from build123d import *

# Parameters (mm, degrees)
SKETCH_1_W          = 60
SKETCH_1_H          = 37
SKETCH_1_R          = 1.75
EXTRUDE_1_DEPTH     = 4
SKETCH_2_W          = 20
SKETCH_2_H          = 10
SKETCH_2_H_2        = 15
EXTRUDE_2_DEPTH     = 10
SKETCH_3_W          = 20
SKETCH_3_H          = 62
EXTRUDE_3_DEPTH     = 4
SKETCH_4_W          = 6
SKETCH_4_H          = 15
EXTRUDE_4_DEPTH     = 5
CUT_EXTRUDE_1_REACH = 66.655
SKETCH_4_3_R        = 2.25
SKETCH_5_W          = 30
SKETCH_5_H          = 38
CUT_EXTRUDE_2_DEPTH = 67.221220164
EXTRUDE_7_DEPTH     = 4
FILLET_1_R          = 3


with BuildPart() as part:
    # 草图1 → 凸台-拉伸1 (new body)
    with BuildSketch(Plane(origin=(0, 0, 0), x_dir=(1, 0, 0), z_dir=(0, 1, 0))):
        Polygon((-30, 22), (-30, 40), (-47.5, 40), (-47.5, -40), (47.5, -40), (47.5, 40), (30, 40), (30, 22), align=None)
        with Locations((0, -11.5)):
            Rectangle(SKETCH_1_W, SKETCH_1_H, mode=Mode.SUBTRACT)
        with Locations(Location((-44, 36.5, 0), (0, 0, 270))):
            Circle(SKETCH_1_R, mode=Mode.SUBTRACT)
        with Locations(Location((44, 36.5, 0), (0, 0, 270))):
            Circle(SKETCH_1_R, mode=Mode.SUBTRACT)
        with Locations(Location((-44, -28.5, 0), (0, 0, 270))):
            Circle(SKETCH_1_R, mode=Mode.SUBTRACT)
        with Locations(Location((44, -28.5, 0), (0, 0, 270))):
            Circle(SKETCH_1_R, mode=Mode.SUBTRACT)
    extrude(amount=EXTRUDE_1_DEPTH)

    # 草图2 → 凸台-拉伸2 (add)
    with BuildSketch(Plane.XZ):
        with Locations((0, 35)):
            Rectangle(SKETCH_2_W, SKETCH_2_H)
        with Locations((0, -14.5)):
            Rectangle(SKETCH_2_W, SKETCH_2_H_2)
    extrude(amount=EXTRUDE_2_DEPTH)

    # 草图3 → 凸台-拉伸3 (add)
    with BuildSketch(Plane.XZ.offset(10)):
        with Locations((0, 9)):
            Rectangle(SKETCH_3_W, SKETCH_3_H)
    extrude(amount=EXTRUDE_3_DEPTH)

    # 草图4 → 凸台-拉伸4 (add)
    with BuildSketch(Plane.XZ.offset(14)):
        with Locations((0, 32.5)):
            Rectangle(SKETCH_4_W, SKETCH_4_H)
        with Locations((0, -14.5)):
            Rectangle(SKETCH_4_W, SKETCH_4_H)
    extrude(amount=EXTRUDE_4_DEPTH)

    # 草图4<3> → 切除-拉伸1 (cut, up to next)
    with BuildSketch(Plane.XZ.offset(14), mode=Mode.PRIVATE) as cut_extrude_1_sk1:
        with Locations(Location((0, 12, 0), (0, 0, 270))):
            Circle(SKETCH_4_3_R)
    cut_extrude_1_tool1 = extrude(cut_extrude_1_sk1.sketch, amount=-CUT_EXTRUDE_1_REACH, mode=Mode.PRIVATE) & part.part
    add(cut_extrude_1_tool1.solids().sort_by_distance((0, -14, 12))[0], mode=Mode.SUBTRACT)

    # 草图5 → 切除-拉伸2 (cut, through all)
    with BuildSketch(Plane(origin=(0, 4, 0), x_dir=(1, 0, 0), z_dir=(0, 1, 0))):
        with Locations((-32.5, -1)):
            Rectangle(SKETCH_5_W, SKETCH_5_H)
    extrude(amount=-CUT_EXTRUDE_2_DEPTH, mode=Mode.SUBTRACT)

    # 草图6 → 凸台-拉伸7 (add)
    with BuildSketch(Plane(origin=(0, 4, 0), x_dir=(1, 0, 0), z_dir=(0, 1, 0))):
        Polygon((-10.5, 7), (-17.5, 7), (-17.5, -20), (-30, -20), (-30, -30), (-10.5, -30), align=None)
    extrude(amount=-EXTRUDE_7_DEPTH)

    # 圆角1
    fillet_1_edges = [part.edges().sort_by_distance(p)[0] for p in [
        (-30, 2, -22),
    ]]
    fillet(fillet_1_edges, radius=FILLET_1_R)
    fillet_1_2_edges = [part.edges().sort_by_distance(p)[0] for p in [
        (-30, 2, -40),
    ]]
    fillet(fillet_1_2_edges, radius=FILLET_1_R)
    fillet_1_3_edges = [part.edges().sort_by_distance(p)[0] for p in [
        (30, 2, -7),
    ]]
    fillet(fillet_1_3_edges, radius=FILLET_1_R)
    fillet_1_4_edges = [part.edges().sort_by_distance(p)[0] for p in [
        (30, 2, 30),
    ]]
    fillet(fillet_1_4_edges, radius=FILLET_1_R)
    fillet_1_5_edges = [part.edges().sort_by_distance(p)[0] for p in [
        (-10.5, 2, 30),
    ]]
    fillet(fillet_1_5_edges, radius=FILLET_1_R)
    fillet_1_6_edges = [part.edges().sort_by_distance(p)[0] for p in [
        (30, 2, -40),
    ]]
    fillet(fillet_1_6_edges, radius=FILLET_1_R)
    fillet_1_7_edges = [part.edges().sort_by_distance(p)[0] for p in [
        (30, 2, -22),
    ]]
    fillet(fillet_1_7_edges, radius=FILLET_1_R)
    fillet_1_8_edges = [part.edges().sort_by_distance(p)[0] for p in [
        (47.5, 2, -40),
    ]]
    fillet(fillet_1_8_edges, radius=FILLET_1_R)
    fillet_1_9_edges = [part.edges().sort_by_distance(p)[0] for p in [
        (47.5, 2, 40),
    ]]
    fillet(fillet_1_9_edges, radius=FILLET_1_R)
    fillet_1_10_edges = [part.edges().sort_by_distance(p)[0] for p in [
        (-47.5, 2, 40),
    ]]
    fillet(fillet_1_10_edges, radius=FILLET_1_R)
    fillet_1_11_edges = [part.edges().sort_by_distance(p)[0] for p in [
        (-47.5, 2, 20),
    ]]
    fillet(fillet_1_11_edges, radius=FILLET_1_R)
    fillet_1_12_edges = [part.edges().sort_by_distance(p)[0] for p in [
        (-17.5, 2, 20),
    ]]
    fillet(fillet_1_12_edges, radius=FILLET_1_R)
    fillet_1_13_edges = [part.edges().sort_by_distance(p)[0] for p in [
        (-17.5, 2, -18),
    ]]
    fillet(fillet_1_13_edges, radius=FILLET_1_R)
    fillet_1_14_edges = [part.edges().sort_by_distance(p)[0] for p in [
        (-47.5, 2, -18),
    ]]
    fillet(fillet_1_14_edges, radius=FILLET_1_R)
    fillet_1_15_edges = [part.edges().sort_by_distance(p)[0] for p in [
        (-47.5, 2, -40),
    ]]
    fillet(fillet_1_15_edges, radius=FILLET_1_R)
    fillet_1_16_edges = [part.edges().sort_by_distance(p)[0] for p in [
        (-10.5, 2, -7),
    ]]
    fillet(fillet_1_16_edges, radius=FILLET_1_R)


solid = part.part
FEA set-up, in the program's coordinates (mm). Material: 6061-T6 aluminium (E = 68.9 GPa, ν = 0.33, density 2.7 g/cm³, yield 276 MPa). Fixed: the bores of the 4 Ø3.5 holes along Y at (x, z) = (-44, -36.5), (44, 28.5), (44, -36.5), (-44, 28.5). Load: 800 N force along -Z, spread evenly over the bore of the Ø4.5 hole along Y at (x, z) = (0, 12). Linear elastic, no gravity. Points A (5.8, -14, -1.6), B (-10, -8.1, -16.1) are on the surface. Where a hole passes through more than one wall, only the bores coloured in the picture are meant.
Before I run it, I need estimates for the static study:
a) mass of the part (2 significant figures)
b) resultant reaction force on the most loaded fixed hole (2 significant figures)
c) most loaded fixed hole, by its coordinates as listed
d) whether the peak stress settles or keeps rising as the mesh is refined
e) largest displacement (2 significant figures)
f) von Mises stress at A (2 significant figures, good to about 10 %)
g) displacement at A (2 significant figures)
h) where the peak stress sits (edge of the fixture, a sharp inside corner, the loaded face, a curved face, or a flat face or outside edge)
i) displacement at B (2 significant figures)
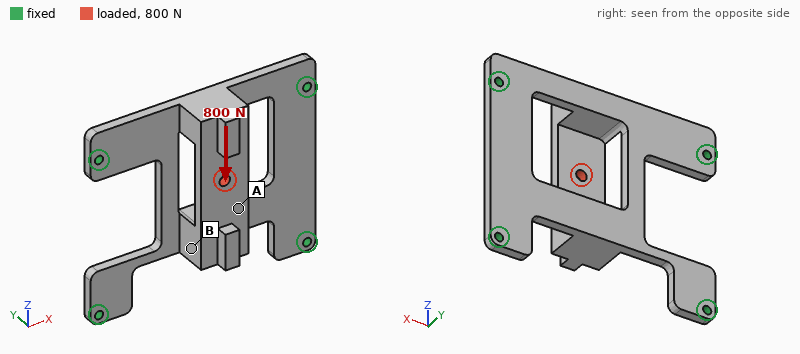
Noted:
71 g
400 N
(44, -36.5)
keeps rising
0.17 mm
20 MPa
0.098 mm
edge of the fixture
0.11 mm
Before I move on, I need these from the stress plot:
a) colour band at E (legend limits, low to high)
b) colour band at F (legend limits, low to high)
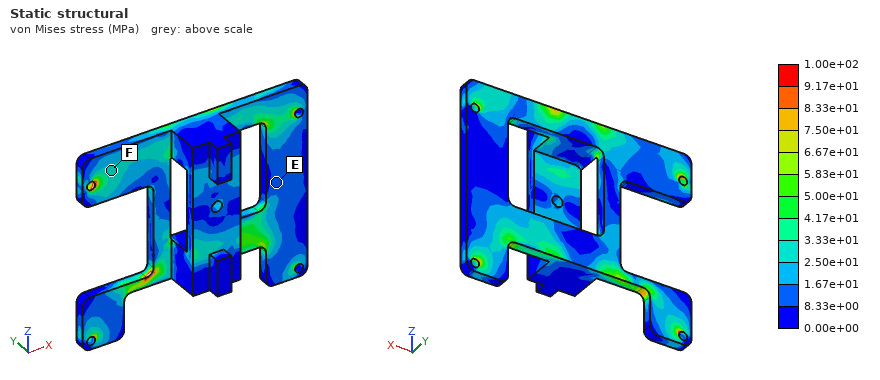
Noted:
8.33e+00 to 1.67e+01 MPa
2.50e+01 to 3.33e+01 MPa
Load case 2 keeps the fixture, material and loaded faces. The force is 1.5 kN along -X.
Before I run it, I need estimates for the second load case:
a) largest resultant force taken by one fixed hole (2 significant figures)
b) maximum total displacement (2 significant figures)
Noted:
560 N
0.16 mm
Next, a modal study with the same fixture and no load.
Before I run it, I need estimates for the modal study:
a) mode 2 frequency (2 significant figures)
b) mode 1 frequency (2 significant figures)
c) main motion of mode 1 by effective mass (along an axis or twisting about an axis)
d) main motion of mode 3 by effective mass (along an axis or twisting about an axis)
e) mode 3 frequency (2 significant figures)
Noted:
1900 Hz
1500 Hz
along Y
along X
3200 Hz
